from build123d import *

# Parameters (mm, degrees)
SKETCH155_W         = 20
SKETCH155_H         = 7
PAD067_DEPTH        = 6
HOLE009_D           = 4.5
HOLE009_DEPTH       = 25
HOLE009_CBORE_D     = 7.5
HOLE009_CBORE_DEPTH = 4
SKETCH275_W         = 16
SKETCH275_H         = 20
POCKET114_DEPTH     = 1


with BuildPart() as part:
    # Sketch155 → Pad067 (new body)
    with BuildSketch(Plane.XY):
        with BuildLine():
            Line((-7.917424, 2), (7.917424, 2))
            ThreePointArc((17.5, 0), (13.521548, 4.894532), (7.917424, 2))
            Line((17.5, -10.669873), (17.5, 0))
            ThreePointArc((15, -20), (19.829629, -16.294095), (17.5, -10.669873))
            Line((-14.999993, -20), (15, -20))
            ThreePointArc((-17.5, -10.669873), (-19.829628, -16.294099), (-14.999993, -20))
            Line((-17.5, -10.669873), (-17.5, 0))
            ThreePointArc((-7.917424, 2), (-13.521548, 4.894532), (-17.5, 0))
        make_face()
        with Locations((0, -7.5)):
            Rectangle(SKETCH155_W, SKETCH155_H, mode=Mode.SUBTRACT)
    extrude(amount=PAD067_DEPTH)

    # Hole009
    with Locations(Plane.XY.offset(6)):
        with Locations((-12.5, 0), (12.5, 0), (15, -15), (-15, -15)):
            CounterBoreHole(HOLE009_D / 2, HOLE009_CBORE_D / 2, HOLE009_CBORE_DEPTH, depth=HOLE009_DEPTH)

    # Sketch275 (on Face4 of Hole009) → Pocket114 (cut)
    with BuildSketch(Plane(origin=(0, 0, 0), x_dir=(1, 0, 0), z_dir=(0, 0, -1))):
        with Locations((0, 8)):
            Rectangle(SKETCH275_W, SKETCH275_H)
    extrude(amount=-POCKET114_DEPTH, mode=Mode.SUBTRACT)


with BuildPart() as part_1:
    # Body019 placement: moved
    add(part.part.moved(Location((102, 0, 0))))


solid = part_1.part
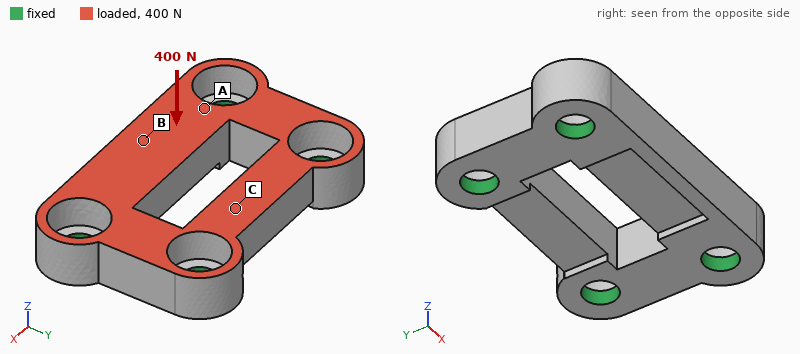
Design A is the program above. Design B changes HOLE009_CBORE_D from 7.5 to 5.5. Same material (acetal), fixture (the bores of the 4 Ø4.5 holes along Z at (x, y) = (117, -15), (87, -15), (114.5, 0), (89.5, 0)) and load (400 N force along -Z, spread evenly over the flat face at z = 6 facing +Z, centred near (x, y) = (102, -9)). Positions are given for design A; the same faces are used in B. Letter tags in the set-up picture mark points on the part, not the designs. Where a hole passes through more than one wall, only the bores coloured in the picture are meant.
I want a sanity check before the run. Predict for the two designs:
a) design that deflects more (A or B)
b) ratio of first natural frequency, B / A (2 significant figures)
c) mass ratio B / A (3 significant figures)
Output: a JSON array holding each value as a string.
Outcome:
["A", "1.1", "1.10"]
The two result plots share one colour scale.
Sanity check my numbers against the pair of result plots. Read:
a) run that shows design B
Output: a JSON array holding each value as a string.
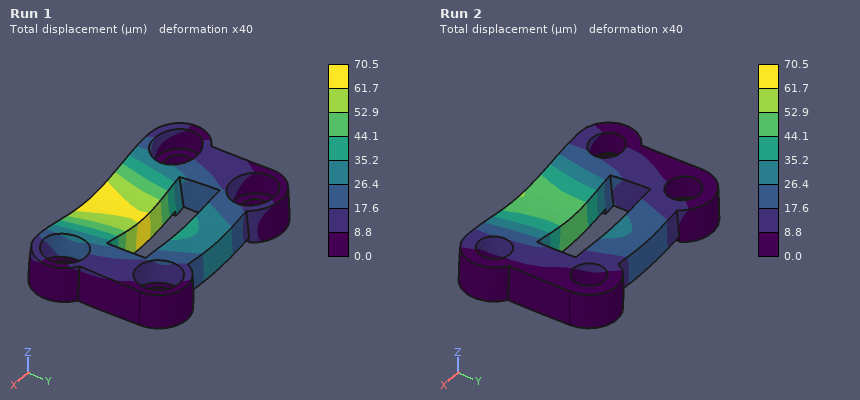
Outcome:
["Run 2"]
